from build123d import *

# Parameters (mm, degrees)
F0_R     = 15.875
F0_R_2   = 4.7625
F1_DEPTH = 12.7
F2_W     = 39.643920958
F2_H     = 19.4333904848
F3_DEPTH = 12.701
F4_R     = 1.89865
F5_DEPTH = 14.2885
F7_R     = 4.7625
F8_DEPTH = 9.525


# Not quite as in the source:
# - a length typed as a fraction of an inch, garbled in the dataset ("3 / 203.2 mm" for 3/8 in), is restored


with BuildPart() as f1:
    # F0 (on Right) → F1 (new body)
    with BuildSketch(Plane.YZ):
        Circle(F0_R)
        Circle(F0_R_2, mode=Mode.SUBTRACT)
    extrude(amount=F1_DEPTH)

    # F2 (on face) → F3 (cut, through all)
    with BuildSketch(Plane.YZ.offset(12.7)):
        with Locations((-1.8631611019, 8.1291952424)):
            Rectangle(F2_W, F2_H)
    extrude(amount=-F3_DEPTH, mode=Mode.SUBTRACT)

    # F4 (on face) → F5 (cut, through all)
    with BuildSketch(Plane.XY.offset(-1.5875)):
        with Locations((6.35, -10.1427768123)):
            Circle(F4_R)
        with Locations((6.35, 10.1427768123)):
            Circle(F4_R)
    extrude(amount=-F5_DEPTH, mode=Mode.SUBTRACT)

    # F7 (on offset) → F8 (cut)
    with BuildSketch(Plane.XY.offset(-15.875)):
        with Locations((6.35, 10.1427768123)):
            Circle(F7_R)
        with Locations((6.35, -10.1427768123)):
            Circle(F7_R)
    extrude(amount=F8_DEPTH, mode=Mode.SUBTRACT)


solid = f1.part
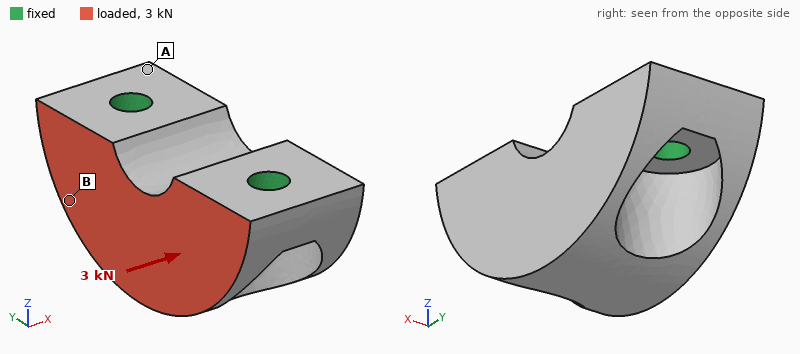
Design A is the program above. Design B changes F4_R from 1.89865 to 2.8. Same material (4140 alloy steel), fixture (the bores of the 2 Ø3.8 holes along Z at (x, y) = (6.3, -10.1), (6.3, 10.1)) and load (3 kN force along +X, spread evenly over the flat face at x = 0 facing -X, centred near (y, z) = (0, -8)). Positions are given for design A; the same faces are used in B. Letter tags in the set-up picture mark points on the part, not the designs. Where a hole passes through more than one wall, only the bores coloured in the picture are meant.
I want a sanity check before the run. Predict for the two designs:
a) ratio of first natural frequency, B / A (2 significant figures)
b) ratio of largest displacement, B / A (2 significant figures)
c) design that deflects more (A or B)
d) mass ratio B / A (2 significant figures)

1.2
0.69
A
0.96
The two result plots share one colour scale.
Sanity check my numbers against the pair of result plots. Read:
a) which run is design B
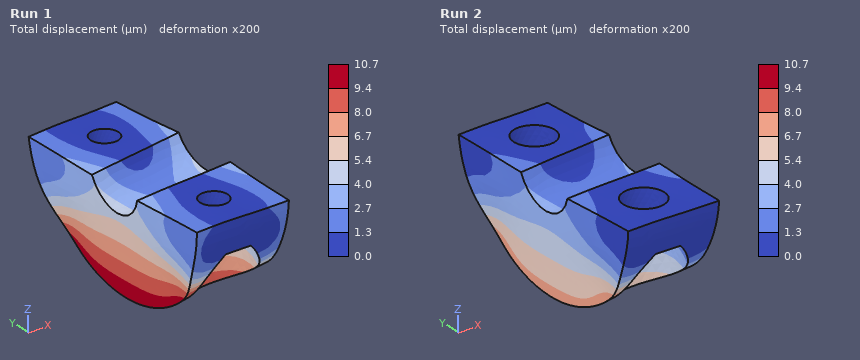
Run 2
